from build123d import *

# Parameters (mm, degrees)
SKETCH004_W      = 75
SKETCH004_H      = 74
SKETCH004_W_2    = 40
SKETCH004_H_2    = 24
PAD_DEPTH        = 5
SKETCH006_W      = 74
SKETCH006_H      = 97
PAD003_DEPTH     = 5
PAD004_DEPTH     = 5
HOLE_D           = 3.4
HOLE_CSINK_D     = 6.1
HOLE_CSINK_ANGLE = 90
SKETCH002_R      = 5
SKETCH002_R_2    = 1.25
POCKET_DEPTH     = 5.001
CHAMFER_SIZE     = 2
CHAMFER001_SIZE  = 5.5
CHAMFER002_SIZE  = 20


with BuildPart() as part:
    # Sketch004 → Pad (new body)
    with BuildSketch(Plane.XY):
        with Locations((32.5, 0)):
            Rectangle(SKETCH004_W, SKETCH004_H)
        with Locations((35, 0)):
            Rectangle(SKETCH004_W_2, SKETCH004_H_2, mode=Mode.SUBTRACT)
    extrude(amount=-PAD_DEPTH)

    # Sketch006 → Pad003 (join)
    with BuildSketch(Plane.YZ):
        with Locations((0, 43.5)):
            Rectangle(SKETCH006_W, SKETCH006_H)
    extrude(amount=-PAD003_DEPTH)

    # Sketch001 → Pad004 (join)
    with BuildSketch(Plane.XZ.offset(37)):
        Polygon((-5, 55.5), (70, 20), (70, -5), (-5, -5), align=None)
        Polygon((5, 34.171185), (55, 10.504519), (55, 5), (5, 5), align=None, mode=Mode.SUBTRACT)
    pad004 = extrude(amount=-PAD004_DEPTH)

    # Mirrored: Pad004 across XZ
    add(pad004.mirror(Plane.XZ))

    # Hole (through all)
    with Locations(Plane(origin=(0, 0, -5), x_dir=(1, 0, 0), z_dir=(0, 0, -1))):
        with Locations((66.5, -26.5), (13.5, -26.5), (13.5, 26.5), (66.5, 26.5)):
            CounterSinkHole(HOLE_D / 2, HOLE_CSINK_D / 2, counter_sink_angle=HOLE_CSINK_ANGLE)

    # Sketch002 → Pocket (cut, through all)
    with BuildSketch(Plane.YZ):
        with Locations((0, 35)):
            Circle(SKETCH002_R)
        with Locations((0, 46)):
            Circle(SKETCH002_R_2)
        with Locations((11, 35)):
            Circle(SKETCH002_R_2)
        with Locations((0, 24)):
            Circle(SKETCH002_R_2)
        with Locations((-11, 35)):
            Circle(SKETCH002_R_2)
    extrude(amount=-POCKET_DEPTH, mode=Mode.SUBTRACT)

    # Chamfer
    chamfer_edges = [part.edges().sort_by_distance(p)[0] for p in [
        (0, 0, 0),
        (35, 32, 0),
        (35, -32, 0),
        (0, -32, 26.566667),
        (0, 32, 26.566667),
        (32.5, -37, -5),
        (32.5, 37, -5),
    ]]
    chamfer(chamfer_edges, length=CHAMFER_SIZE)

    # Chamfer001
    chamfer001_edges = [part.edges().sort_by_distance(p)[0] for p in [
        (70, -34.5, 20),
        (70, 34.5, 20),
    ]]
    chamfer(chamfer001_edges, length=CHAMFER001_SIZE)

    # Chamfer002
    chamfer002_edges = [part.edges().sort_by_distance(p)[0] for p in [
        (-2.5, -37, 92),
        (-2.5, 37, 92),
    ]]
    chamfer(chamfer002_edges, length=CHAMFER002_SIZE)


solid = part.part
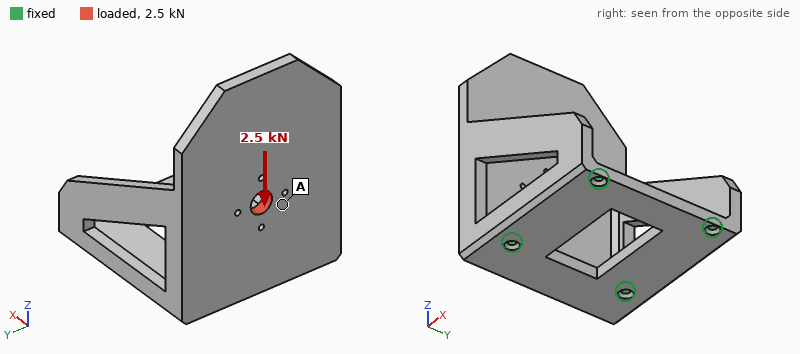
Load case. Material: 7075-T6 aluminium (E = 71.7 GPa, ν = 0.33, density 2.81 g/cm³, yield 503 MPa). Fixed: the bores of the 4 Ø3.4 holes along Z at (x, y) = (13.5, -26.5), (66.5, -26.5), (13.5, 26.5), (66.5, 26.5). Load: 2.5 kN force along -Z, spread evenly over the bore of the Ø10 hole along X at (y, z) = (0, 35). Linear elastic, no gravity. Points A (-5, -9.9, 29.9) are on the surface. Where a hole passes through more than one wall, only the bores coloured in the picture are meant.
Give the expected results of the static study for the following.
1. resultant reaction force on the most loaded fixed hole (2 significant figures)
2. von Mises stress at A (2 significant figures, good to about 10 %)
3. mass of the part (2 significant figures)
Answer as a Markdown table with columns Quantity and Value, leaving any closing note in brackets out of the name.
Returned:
| Quantity | Value |
|---|---|
| resultant reaction force on the most loaded fixed hole | 1.6 kN |
| von Mises stress at A | 10.0 MPa |
| mass of the part | 200 g |
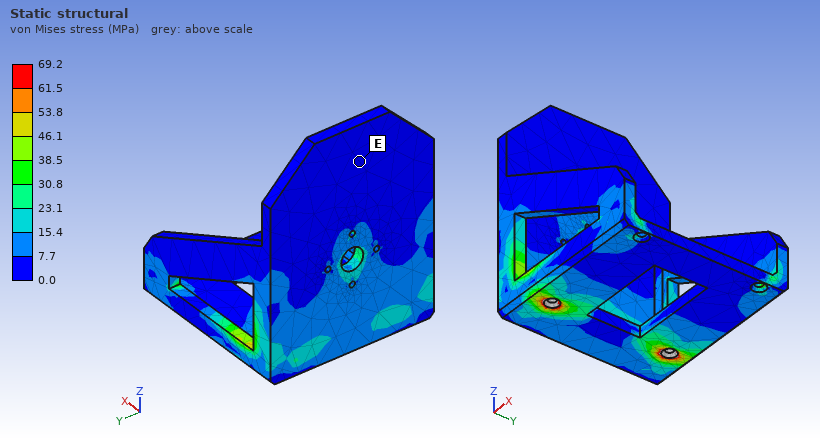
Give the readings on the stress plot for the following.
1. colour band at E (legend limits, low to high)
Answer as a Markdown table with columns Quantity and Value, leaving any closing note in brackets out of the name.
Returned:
| Quantity | Value |
|---|---|
| colour band at E | 0.0 to 7.7 MPa |
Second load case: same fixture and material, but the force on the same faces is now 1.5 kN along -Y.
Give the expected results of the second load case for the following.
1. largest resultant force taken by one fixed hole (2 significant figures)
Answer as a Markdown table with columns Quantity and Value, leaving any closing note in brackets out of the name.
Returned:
| Quantity | Value |
|---|---|
| largest resultant force taken by one fixed hole | 1.4 kN |
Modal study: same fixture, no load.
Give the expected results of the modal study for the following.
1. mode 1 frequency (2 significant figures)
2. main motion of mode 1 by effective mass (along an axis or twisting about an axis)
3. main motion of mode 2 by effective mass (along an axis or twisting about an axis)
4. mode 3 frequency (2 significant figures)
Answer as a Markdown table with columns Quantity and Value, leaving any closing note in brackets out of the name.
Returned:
| Quantity | Value |
|---|---|
| mode 1 frequency | 1400 Hz |
| main motion of mode 1 by effective mass | along X |
| main motion of mode 2 by effective mass | along Y |
| mode 3 frequency | 2900 Hz |
